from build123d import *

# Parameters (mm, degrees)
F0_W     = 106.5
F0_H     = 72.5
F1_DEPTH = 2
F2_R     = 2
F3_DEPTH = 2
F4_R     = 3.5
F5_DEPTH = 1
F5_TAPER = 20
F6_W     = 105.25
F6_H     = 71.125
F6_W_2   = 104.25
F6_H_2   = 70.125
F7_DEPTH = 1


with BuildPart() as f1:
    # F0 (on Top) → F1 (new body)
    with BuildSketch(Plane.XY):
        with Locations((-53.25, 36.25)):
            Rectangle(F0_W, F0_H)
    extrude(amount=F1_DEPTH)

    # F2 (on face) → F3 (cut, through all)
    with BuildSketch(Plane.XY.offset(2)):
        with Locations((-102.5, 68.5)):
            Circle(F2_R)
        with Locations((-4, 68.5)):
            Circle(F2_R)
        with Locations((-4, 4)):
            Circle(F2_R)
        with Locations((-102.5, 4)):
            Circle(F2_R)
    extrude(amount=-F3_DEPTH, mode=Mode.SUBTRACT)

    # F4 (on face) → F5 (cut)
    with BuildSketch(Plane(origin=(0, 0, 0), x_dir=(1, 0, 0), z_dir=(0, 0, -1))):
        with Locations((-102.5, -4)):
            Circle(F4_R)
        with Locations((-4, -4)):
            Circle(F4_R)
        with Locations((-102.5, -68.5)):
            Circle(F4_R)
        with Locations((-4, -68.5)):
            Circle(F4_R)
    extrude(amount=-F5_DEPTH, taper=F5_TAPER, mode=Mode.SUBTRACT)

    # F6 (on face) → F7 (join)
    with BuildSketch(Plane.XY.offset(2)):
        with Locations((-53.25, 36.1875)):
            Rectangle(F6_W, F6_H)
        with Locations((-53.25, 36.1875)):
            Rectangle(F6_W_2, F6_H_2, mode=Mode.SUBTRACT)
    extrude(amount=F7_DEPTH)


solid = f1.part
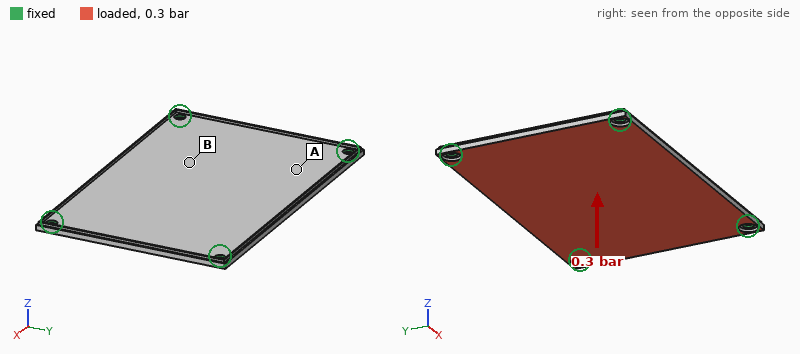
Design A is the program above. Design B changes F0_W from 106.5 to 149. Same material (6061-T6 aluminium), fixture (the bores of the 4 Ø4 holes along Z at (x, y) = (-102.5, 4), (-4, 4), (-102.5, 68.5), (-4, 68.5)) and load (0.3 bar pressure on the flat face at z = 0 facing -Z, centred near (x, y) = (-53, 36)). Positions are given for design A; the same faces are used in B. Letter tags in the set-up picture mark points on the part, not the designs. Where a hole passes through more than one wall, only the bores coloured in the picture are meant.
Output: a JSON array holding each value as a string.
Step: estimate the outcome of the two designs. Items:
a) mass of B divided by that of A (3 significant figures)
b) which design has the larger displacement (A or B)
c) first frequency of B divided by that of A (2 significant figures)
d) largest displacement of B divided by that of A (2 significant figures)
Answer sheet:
["1.40", "A", "1.0", "0.84"]
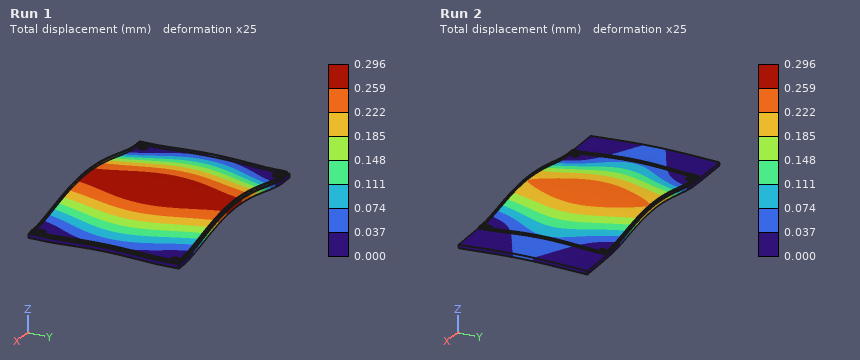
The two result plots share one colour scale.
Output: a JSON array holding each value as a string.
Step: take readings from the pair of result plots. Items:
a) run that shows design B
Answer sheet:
["Run 2"]
